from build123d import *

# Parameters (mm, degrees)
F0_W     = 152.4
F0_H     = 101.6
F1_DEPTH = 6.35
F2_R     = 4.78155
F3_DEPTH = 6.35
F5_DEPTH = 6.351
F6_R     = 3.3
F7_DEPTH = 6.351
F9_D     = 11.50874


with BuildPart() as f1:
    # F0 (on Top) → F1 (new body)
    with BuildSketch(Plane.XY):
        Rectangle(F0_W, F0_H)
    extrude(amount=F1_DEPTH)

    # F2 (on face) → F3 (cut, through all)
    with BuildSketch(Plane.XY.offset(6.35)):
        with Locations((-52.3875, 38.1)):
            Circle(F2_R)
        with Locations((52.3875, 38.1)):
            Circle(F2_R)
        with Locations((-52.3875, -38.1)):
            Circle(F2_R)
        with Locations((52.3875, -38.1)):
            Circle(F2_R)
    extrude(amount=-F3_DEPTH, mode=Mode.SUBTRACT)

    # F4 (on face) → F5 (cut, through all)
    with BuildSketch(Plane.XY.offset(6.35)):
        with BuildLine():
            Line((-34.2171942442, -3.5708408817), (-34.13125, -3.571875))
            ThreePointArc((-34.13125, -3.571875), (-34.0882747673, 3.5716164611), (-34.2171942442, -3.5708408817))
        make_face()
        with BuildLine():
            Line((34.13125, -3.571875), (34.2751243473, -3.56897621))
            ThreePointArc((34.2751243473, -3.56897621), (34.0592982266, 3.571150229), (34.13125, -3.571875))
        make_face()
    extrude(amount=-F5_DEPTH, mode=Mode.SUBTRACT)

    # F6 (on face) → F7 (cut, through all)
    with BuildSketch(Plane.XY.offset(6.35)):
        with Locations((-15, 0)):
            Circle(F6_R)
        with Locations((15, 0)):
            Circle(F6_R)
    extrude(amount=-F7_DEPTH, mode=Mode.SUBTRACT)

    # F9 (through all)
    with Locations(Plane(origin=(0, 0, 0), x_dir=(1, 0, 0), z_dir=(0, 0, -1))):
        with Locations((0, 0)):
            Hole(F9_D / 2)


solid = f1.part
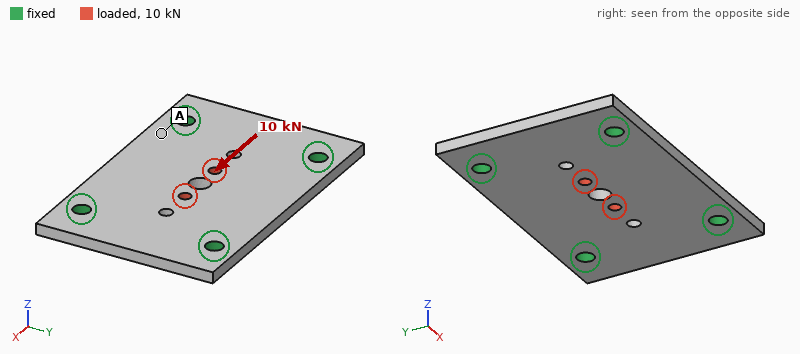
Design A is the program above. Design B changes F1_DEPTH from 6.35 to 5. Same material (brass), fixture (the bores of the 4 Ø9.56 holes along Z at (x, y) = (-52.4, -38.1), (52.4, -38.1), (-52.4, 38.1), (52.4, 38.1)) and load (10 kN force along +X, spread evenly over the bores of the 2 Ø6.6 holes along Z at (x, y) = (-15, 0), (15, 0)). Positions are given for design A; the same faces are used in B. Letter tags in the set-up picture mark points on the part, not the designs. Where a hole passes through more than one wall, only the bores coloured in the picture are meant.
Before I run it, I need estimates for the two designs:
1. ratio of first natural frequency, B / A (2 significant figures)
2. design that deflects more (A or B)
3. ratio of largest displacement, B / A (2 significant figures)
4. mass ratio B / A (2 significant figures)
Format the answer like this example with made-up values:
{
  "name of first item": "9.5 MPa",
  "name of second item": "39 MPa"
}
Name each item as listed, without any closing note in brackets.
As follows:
{
  "ratio of first natural frequency, B / A": "0.81",
  "design that deflects more": "B",
  "ratio of largest displacement, B / A": "1.3",
  "mass ratio B / A": "0.79"
}
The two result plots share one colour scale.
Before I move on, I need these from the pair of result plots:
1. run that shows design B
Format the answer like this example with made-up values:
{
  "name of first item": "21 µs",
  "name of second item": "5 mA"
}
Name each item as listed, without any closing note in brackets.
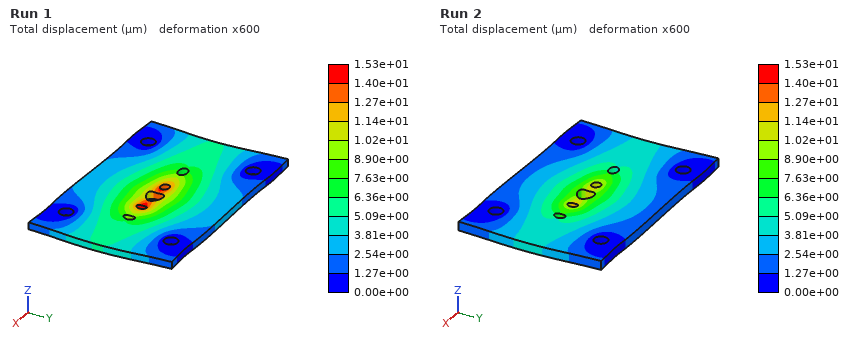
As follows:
{
  "run that shows design B": "Run 1"
}
